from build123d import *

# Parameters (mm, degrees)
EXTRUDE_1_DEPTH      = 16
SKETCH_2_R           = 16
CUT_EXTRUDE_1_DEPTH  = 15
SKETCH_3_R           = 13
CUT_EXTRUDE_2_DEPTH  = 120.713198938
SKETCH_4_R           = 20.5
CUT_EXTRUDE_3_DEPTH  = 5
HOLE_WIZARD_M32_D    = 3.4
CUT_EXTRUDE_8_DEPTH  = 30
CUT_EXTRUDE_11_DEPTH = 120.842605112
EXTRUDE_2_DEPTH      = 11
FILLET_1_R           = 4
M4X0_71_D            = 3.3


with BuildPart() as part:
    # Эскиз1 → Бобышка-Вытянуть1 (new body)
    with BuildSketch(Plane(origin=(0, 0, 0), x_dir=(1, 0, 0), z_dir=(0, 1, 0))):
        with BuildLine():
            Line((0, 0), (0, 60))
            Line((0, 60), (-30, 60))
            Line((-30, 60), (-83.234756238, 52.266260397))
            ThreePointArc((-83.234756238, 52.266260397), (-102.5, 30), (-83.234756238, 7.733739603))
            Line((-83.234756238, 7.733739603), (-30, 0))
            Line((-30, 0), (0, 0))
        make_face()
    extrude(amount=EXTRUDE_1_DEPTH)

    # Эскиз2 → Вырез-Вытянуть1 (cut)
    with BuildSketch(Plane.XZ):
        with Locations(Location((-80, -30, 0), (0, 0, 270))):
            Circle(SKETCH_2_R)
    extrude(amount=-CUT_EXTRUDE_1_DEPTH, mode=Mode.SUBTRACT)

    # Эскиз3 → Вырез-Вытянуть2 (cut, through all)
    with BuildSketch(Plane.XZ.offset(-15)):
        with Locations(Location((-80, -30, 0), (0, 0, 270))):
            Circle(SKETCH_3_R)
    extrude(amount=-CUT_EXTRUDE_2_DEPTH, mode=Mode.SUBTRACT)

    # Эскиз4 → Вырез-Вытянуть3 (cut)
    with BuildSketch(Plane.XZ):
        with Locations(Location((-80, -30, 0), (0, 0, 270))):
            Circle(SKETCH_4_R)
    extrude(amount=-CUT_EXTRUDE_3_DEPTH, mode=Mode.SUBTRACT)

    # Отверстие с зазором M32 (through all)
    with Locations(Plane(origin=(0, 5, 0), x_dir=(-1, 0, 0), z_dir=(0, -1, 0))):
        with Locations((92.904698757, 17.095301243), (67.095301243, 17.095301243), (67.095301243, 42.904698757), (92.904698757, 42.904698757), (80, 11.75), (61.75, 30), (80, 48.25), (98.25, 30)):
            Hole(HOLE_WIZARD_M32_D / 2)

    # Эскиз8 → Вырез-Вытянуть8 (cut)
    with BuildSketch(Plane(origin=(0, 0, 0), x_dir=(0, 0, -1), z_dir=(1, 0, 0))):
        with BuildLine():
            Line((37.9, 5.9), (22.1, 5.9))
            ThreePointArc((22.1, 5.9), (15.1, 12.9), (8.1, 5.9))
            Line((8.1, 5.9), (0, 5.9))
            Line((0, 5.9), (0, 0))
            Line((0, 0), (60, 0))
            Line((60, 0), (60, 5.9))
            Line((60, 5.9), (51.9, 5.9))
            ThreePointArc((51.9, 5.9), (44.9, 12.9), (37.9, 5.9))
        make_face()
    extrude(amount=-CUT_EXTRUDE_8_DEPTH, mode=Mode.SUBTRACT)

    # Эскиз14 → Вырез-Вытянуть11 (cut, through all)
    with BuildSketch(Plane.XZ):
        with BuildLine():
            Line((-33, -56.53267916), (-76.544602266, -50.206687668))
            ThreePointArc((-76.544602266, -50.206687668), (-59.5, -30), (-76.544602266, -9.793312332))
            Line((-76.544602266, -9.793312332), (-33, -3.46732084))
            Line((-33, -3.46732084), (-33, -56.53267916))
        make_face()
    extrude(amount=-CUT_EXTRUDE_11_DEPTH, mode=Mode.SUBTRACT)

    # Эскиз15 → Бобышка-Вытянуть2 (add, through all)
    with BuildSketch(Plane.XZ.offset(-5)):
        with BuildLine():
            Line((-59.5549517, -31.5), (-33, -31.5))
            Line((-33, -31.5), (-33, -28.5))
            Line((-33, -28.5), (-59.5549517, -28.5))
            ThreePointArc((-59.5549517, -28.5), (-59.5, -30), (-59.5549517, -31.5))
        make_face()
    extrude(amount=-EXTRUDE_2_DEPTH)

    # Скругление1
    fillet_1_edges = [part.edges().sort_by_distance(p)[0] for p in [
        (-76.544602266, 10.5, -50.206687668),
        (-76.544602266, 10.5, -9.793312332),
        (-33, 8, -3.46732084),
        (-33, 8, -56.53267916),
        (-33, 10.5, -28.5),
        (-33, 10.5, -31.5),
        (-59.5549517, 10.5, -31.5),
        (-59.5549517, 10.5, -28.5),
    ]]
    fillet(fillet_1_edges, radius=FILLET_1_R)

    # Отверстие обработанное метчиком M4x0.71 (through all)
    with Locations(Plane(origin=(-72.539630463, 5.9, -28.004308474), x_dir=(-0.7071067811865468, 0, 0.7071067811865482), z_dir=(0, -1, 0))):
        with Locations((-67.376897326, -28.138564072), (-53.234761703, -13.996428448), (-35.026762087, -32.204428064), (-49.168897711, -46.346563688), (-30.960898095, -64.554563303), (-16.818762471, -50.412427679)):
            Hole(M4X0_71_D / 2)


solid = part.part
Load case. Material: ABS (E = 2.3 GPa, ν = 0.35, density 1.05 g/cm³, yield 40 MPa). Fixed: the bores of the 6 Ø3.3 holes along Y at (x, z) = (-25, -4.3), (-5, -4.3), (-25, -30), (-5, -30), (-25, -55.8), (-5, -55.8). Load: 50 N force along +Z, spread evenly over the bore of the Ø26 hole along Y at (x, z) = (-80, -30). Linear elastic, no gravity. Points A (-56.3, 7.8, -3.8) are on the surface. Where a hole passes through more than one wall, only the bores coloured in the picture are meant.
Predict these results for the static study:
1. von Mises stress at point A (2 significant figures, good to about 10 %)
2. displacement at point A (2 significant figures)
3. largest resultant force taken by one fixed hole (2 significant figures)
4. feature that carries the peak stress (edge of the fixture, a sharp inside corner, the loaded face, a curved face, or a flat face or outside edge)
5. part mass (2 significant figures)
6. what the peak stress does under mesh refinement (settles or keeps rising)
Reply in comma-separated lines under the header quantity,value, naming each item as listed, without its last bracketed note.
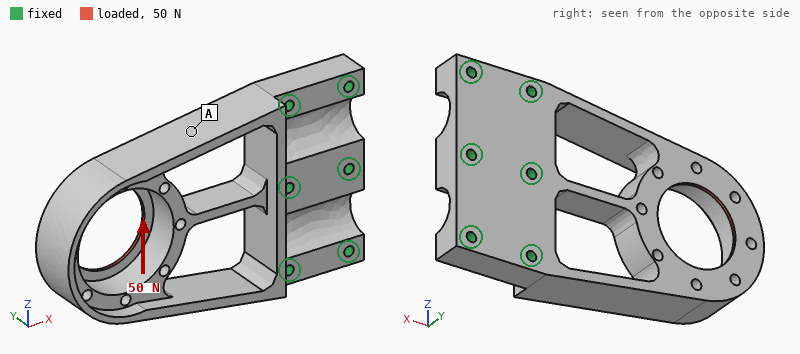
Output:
quantity,value
von Mises stress at point A,1.6 MPa
displacement at point A,0.31 mm
largest resultant force taken by one fixed hole,46 N
feature that carries the peak stress,a sharp inside corner
part mass,31 g
what the peak stress does under mesh refinement,keeps rising
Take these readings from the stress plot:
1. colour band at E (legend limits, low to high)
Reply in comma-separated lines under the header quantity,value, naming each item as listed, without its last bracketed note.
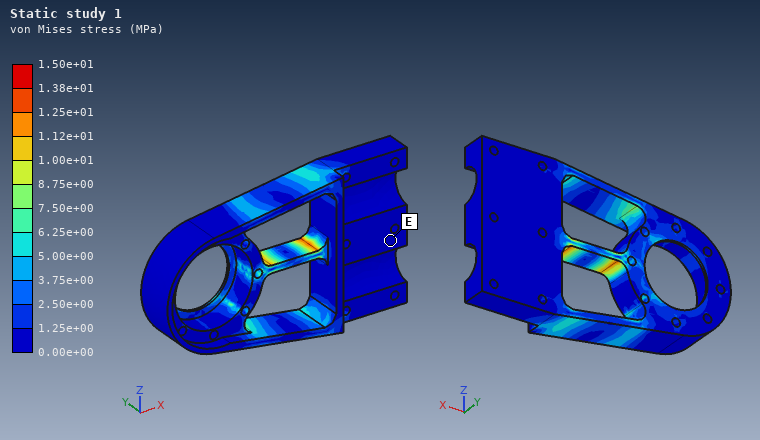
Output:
quantity,value
colour band at E,0.00e+00 to 1.25e+00 MPa
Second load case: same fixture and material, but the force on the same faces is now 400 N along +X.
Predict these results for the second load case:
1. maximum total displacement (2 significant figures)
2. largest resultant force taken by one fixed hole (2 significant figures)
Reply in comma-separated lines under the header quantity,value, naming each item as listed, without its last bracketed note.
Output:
quantity,value
maximum total displacement,1.3 mm
largest resultant force taken by one fixed hole,130 N
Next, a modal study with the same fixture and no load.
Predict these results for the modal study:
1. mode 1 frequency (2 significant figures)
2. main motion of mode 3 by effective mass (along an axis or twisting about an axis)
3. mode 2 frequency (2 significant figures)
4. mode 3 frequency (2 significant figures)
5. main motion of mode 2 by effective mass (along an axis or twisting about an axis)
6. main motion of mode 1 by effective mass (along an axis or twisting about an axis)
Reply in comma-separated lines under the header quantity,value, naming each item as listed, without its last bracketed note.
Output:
quantity,value
mode 1 frequency,420 Hz
main motion of mode 3 by effective mass,twisting about X
mode 2 frequency,520 Hz
mode 3 frequency,960 Hz
main motion of mode 2 by effective mass,along Z
main motion of mode 1 by effective mass,along Y
